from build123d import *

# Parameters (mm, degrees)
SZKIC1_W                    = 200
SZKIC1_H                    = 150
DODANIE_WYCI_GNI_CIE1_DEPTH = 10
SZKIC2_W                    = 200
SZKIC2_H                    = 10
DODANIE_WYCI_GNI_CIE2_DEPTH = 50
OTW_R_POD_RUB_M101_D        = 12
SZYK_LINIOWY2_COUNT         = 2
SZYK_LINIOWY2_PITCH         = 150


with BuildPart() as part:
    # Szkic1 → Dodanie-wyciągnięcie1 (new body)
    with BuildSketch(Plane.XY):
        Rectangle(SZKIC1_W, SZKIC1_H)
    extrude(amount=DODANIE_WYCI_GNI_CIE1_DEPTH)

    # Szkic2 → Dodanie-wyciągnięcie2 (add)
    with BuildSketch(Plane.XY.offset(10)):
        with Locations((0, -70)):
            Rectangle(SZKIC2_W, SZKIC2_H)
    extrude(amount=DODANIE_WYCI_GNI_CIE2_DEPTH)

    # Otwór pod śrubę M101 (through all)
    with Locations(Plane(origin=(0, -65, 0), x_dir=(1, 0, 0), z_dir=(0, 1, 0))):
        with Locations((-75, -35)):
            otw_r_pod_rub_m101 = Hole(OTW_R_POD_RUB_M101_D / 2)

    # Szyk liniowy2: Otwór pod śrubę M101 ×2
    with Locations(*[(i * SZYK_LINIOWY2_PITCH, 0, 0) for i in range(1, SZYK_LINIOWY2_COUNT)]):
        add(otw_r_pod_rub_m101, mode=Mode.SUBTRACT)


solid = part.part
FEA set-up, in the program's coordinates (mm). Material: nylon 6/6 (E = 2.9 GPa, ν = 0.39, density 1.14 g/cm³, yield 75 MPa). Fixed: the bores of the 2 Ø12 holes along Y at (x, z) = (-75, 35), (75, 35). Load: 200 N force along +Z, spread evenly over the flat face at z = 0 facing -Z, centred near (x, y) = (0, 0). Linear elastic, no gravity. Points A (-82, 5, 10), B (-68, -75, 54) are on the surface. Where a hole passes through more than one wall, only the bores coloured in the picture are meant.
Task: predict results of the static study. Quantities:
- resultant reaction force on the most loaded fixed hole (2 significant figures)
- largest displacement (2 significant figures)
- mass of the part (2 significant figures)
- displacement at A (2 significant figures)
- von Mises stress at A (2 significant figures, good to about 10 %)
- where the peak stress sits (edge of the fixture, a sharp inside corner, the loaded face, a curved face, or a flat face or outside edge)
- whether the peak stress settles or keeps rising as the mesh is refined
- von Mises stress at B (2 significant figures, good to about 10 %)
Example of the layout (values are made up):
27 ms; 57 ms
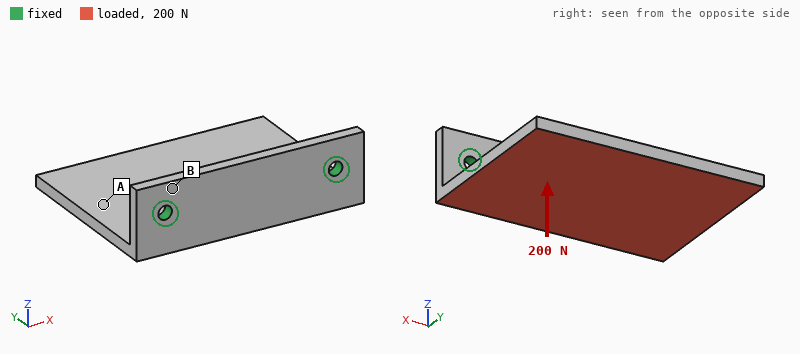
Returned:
110 N; 2.8 mm; 450 g; 1.2 mm; 0.93 MPa; edge of the fixture; keeps rising; 2.4 MPa
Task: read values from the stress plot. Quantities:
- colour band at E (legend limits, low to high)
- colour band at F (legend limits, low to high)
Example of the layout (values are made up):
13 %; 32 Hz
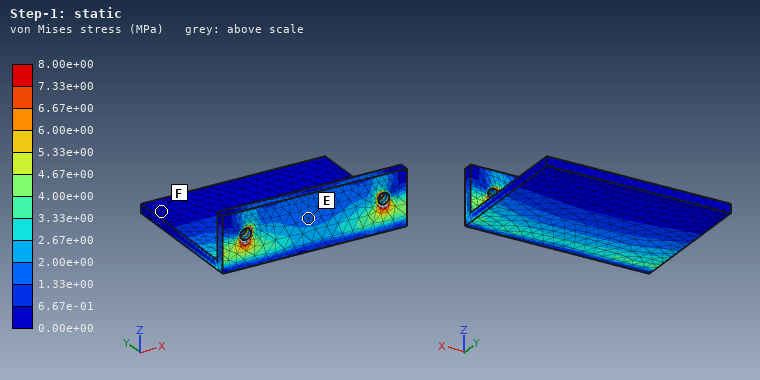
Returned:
1.33e+00 to 2.00e+00 MPa; 0.00e+00 to 6.67e-01 MPa
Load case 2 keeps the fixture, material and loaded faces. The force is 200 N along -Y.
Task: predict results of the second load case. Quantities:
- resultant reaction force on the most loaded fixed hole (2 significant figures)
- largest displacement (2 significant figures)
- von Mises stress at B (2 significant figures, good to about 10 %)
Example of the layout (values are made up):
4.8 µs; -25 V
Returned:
100 N; 0.59 mm; 0.58 MPa
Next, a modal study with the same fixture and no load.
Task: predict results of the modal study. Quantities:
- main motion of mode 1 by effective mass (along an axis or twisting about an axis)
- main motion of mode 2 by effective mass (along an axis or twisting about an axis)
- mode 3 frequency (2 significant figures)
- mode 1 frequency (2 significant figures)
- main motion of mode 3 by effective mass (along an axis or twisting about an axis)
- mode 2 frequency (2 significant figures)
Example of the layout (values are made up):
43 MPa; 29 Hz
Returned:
along Z; twisting about Y; 450 Hz; 90 Hz; along X; 200 Hz
